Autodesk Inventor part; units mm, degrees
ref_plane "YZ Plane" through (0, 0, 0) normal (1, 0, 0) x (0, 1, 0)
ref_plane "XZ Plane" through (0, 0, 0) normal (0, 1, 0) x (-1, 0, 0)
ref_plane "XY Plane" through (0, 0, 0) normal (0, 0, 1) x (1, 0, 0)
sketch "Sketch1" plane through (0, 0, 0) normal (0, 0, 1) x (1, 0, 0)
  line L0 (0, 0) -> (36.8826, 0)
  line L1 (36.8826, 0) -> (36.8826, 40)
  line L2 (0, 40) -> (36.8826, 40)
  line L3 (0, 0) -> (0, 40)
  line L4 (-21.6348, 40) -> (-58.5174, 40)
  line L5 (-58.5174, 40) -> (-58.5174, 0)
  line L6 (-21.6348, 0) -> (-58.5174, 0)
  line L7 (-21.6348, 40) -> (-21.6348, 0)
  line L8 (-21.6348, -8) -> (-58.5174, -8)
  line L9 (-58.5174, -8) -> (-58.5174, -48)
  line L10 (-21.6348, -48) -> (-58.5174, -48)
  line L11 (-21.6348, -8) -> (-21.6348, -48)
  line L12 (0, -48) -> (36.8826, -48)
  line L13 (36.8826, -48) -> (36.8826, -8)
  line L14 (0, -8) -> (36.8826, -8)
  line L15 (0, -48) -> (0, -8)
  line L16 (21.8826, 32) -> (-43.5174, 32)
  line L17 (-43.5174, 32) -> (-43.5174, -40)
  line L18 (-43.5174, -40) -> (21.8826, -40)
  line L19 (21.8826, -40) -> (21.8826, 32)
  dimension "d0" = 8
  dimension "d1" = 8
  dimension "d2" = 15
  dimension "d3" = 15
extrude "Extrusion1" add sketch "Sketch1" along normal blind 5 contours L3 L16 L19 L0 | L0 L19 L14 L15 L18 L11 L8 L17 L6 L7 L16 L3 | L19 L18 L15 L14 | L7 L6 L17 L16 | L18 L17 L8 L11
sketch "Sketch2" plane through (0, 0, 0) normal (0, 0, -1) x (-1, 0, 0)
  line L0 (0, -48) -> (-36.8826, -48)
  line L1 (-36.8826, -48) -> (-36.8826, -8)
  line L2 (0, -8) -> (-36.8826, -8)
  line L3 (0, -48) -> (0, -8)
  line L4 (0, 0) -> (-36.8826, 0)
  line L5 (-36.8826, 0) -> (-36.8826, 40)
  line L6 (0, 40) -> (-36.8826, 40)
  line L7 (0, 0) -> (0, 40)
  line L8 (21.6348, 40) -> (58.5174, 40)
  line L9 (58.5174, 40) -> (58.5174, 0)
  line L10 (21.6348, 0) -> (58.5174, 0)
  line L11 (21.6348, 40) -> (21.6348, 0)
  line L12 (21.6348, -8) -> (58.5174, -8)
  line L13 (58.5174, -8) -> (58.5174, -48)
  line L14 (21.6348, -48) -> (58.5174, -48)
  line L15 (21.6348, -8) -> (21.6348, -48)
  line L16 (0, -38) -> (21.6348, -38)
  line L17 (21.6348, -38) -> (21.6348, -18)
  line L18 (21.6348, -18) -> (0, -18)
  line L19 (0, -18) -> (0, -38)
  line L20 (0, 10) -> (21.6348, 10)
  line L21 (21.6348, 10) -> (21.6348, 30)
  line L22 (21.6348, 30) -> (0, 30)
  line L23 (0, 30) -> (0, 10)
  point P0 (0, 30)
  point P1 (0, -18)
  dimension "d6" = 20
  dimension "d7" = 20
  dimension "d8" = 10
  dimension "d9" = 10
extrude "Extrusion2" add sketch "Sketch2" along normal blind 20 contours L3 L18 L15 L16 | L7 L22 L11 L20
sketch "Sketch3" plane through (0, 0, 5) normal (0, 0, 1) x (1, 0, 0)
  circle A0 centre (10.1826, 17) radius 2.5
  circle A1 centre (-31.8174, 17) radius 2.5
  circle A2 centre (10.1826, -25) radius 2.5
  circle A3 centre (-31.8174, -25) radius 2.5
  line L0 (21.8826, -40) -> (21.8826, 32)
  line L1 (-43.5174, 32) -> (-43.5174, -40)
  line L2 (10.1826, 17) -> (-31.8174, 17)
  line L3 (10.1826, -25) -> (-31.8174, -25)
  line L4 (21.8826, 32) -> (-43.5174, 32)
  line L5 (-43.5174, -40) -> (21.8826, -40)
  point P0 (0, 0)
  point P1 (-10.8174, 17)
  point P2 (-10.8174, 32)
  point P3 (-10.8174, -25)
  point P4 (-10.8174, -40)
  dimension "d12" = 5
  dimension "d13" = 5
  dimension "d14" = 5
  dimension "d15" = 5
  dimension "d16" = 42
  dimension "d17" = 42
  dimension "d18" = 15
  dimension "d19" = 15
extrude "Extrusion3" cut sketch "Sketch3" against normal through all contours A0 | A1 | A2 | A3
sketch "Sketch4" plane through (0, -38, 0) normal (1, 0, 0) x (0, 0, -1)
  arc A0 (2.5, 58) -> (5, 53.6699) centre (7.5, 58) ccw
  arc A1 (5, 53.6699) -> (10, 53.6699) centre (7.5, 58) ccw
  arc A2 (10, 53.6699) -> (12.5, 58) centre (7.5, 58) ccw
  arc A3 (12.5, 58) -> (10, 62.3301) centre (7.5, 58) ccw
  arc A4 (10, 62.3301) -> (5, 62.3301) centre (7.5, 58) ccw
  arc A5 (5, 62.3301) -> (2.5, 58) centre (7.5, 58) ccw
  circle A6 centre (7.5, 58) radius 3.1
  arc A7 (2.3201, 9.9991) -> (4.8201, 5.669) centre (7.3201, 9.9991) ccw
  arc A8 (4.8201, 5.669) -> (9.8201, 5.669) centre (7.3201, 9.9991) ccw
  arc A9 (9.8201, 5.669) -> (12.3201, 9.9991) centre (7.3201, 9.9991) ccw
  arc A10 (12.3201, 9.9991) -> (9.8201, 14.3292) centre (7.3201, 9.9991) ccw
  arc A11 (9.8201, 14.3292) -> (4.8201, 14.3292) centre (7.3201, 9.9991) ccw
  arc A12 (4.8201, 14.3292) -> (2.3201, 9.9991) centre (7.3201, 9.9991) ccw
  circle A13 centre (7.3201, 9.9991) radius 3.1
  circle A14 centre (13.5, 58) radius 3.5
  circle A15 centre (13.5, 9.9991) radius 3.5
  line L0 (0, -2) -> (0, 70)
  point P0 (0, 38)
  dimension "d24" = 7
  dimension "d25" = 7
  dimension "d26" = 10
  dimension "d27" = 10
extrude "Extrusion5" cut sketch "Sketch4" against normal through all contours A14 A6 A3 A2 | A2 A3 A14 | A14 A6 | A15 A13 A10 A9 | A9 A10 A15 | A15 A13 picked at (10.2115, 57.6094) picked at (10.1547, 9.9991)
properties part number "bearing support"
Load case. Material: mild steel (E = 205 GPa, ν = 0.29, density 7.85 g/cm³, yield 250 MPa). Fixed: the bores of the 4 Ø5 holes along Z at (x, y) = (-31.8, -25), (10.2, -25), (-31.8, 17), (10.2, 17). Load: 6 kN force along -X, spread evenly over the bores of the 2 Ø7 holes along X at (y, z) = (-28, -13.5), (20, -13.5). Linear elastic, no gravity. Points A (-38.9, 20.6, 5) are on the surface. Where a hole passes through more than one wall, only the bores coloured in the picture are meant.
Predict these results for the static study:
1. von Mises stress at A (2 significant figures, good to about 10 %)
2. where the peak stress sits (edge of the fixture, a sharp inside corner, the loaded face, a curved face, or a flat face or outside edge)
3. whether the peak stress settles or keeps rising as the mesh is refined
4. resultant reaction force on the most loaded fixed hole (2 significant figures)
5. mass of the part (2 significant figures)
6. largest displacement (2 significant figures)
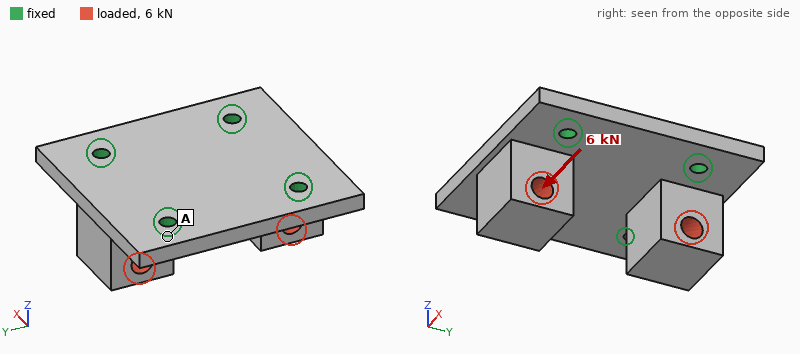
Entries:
17 MPa
edge of the fixture
keeps rising
2.1 kN
300 g
15 µm
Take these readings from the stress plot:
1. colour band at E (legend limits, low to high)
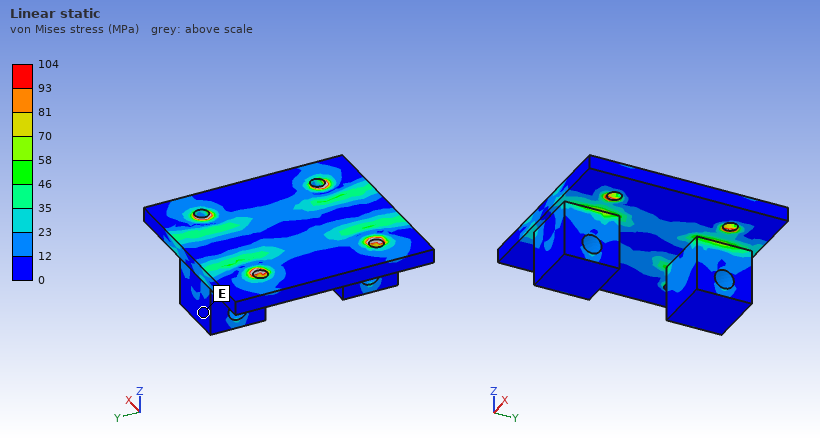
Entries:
0 to 12 MPa
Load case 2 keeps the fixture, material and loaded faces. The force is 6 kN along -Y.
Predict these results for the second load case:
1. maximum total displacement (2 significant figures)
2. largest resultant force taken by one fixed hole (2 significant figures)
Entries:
45 µm
1.7 kN
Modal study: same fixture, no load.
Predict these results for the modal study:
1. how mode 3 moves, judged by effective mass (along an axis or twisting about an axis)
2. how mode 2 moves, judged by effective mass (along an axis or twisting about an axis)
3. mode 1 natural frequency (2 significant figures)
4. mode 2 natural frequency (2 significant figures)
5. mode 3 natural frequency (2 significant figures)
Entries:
along Z
along Y
5600 Hz
6400 Hz
9700 Hz
